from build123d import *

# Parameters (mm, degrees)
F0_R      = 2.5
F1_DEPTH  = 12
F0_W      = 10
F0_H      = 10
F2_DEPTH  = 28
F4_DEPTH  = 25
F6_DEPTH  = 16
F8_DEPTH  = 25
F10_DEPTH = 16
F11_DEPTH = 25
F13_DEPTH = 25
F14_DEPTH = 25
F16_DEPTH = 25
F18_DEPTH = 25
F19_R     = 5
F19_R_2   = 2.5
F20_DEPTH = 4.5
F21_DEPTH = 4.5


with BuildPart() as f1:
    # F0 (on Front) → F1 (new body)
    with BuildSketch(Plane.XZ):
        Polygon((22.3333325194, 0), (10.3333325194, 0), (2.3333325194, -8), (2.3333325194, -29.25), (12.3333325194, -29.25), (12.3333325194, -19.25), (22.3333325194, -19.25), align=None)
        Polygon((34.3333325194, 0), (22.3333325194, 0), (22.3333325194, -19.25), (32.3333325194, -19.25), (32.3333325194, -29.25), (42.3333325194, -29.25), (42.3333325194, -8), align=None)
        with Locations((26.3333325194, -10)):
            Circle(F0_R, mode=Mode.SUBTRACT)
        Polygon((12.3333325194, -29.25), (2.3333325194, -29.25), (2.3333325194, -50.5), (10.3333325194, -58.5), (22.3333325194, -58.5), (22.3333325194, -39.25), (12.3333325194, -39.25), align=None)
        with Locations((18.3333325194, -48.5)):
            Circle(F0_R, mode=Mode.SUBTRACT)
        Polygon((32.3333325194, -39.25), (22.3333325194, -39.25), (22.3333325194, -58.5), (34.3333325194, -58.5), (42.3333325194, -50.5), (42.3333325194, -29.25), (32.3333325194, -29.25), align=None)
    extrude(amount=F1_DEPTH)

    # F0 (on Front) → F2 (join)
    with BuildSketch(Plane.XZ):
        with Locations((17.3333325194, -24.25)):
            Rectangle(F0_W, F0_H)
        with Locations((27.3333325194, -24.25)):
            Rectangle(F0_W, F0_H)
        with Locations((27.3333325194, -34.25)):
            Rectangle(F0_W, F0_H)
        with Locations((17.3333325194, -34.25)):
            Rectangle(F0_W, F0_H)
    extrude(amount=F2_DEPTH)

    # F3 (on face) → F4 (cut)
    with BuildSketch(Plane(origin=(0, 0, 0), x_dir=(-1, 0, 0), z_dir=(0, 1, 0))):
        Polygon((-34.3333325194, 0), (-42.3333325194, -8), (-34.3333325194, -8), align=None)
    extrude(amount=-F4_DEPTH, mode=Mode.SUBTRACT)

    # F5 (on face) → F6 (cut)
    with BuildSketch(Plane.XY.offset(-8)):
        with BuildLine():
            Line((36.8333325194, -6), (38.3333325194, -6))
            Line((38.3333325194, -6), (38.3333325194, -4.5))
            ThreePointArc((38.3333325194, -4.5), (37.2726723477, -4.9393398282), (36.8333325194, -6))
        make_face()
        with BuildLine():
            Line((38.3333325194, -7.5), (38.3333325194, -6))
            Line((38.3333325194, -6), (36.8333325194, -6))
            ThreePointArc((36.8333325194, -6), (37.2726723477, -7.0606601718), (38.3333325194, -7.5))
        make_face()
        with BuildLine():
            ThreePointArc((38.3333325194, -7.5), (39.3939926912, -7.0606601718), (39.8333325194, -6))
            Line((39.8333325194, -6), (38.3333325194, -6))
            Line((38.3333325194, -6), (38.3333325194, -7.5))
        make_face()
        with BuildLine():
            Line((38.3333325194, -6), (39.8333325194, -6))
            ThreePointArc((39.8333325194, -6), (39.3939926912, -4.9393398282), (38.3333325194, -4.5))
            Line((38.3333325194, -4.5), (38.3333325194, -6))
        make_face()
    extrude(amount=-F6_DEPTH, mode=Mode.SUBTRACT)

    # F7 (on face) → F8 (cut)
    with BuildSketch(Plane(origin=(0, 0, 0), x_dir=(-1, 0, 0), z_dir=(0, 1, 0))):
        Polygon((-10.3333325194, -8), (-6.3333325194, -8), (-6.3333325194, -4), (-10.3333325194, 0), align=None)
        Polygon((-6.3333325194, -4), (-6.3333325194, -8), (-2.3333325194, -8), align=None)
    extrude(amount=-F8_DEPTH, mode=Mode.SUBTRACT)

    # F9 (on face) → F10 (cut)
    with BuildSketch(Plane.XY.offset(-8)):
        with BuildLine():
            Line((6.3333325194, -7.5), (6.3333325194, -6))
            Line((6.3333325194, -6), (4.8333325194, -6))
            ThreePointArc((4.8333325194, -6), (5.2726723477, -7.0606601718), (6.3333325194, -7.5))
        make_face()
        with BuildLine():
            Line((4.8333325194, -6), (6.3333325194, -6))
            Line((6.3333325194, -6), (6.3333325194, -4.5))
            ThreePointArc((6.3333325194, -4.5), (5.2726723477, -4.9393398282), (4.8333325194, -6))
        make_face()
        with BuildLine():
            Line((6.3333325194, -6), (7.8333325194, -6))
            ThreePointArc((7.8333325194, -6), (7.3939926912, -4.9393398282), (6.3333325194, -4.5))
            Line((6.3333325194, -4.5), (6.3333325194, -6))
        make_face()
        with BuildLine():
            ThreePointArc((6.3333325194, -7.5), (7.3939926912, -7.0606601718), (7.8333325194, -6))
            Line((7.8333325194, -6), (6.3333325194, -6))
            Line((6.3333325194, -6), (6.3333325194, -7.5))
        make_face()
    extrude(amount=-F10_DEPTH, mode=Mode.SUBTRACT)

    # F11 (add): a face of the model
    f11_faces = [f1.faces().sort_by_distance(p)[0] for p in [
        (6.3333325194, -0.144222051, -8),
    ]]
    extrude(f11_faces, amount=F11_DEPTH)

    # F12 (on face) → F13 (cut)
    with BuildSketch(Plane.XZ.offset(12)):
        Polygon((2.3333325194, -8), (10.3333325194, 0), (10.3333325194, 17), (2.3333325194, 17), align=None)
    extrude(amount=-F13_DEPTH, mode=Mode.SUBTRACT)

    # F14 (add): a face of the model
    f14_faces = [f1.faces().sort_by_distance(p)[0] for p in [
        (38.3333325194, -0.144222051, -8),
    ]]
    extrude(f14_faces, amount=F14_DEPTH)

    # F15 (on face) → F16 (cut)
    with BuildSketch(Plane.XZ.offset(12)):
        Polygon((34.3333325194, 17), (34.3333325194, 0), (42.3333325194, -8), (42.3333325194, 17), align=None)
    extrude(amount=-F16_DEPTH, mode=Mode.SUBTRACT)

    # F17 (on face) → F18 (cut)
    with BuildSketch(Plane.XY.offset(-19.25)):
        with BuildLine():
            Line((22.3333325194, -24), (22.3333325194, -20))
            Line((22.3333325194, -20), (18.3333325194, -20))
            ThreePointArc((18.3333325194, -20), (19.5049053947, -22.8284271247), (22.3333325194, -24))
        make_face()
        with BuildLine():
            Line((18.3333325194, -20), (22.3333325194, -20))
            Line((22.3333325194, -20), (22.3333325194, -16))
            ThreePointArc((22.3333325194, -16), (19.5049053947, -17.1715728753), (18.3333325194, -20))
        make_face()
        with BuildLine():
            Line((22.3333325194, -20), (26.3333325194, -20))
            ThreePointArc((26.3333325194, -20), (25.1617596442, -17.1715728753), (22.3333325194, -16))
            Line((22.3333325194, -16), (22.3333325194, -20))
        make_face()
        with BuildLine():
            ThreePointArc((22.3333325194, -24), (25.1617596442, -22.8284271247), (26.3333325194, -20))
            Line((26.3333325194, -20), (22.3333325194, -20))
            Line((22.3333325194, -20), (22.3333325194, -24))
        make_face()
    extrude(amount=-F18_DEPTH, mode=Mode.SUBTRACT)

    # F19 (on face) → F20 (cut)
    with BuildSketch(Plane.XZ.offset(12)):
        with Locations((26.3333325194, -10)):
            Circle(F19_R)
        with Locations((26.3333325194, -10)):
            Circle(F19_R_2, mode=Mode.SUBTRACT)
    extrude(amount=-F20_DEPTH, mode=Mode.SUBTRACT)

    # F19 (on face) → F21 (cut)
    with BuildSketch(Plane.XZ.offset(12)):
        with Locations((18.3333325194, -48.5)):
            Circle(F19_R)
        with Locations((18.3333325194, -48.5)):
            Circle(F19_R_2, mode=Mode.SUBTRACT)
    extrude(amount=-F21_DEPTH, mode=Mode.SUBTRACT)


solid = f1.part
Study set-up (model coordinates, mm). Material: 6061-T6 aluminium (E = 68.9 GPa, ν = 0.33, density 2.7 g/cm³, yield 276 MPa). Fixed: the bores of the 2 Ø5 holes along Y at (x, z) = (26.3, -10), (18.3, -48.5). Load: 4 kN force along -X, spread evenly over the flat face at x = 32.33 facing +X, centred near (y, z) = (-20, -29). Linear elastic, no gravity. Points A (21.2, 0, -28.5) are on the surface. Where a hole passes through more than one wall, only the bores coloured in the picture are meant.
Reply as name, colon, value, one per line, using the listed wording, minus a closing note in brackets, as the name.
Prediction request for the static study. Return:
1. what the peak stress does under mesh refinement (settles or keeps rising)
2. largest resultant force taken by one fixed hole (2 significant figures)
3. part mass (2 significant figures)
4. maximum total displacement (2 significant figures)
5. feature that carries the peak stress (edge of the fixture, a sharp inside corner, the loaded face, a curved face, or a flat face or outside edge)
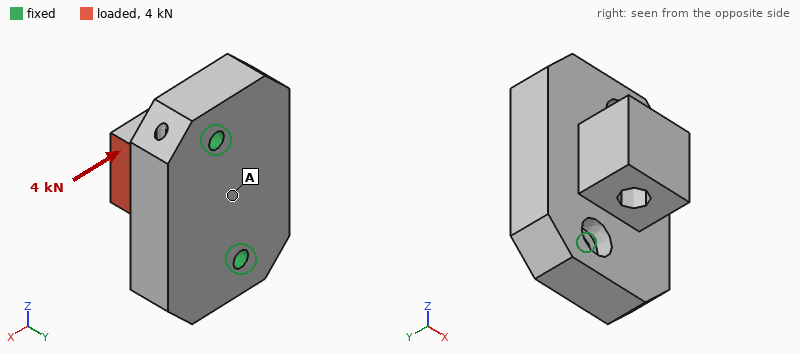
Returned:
what the peak stress does under mesh refinement: keeps rising
largest resultant force taken by one fixed hole: 2.0 kN
part mass: 83 g
maximum total displacement: 79 µm
feature that carries the peak stress: edge of the fixture
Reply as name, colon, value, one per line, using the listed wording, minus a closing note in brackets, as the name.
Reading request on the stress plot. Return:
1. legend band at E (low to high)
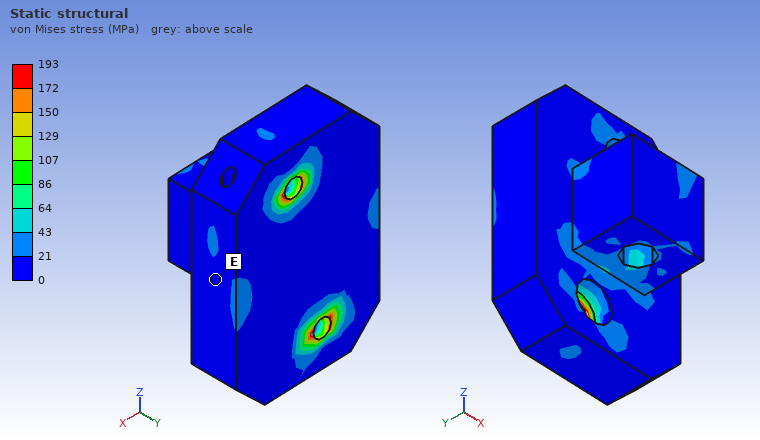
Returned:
legend band at E: 0 to 21 MPa
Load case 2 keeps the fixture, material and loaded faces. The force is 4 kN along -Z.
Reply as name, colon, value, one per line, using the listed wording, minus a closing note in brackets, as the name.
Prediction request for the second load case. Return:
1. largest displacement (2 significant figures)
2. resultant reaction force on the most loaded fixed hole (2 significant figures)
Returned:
largest displacement: 40 µm
resultant reaction force on the most loaded fixed hole: 2.9 kN
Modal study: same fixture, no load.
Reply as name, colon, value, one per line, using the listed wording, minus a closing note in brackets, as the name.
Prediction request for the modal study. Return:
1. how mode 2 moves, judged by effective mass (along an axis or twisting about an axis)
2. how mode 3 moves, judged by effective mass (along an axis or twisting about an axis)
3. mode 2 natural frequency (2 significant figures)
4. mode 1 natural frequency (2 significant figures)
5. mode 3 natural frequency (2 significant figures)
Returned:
how mode 2 moves, judged by effective mass: along Y
how mode 3 moves, judged by effective mass: along Z
mode 2 natural frequency: 14 kHz
mode 1 natural frequency: 7100 Hz
mode 3 natural frequency: 19 kHz
